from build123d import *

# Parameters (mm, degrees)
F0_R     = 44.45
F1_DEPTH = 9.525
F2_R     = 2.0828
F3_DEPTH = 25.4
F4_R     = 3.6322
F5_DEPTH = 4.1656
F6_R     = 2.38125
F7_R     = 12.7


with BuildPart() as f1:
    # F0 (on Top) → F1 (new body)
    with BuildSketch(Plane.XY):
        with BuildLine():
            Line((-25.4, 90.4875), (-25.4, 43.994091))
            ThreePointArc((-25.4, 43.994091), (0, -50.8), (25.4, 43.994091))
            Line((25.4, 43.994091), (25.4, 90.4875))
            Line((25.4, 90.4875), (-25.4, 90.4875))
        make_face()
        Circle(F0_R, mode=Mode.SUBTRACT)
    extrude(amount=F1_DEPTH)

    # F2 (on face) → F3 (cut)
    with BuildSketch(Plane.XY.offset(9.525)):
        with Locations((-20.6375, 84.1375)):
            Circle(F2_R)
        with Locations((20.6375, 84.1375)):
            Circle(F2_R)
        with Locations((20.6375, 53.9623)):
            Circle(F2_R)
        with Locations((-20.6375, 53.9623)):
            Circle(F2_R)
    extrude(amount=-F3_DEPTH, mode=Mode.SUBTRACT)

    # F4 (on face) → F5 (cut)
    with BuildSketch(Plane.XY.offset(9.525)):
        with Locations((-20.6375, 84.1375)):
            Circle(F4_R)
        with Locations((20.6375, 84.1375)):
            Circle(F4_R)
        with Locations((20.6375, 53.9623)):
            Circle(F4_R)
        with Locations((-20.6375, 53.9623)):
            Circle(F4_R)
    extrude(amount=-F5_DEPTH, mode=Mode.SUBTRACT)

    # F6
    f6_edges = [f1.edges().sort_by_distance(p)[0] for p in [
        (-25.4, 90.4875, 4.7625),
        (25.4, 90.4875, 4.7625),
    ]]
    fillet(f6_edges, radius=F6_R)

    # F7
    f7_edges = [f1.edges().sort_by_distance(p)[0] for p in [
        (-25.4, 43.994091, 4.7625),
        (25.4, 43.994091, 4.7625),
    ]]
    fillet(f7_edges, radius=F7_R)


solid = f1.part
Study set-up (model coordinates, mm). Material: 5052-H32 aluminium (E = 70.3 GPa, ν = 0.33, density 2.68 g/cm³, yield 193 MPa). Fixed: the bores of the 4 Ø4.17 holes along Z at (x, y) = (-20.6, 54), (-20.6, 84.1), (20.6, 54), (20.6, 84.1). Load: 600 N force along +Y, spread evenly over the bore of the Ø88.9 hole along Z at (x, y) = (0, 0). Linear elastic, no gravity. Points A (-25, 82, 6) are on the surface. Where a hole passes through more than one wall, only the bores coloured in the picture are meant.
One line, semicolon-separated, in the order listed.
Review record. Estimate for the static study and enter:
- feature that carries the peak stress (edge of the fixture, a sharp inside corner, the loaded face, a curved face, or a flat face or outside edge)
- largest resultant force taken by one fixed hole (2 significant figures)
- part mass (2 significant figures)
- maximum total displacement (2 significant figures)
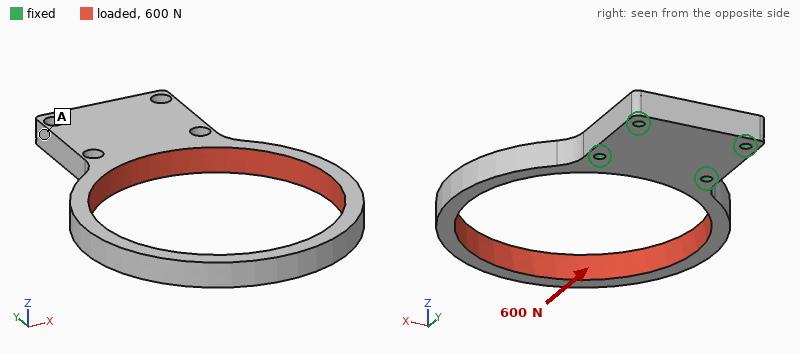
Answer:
a curved face; 350 N; 100 g; 0.12 mm
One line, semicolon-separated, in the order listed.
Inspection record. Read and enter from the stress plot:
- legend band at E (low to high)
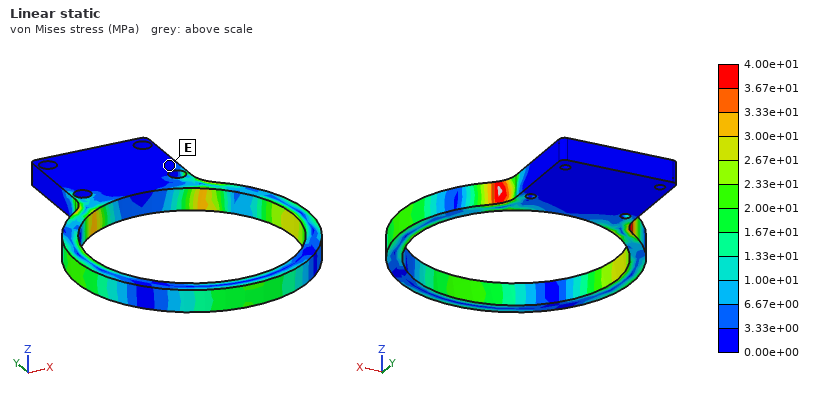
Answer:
0.00e+00 to 3.33e+00 MPa
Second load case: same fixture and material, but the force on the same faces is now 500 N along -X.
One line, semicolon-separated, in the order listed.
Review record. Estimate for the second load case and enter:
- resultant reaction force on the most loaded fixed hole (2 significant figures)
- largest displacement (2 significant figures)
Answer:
650 N; 0.78 mm
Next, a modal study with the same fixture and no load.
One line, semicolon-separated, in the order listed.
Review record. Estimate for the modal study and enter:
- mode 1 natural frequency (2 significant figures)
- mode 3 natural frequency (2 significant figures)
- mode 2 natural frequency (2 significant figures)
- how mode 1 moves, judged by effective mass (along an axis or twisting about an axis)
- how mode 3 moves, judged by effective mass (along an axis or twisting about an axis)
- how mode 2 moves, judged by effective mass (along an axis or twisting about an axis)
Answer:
460 Hz; 1200 Hz; 620 Hz; along Z; twisting about Y; along X
